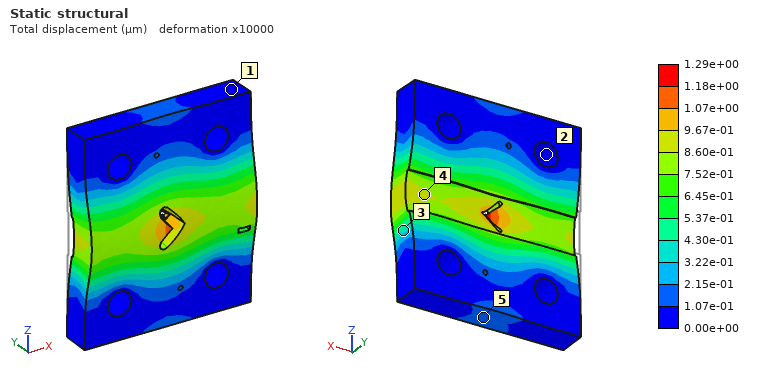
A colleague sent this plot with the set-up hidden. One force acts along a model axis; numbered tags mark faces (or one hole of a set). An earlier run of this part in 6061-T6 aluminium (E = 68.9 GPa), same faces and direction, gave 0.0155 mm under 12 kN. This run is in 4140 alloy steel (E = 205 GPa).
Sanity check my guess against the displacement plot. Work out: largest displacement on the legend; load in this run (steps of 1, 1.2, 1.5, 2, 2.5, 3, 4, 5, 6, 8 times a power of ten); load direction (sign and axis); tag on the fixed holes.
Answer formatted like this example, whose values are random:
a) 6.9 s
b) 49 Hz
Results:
a) 1.29e+00 µm
b) 3 kN
c) -Y
d) 2
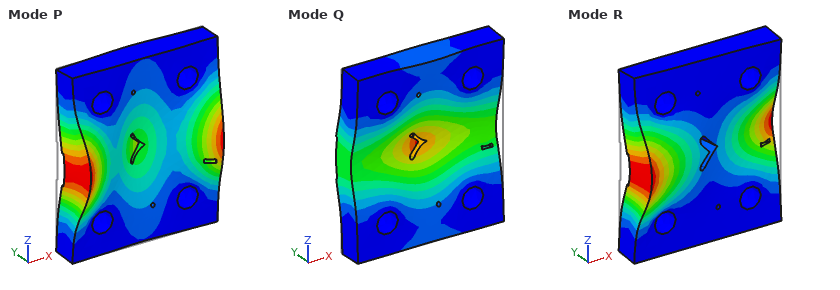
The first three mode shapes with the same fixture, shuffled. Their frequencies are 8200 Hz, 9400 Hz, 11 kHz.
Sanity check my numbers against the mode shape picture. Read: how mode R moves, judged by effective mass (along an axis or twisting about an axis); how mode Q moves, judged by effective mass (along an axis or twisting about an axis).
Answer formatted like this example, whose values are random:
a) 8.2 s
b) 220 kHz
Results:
a) twisting about Z
b) along Y
